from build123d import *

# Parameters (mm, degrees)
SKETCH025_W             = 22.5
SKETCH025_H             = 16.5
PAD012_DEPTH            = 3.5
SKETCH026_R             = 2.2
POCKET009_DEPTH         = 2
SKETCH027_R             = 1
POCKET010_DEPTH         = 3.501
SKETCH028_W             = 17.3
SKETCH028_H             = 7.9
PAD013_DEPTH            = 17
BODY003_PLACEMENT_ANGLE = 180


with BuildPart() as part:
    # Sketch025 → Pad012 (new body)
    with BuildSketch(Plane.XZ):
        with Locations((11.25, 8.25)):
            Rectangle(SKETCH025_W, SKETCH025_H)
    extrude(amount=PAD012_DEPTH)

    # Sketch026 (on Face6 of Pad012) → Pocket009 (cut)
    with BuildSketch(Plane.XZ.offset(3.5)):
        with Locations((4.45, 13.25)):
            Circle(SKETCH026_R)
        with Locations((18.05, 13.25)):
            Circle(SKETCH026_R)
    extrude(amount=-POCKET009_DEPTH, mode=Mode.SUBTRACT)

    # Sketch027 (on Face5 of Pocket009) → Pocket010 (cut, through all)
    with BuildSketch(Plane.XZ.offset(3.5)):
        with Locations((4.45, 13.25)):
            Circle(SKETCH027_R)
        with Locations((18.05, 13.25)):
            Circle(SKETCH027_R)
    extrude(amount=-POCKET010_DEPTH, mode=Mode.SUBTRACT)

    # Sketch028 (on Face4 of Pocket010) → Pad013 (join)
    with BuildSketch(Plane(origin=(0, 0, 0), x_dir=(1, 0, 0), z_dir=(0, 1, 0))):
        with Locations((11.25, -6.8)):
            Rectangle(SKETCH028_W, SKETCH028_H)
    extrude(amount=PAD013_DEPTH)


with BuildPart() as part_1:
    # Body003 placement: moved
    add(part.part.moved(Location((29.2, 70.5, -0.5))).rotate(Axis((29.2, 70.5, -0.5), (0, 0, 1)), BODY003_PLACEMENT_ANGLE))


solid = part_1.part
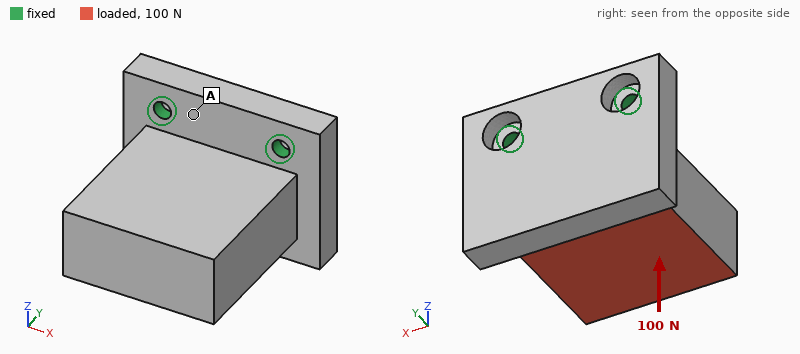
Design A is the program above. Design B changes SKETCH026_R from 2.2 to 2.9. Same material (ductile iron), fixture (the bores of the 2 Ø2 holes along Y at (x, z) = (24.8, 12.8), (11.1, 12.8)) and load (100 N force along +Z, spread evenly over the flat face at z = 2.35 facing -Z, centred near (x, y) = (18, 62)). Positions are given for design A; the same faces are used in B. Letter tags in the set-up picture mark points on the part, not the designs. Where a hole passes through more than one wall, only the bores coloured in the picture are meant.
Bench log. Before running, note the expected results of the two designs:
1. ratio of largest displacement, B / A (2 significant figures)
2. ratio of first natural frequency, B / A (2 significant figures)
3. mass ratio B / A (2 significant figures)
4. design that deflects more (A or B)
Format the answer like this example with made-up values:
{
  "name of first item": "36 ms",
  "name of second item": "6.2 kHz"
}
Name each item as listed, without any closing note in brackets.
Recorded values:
{
  "ratio of largest displacement, B / A": "1.1",
  "ratio of first natural frequency, B / A": "0.94",
  "mass ratio B / A": "0.99",
  "design that deflects more": "B"
}
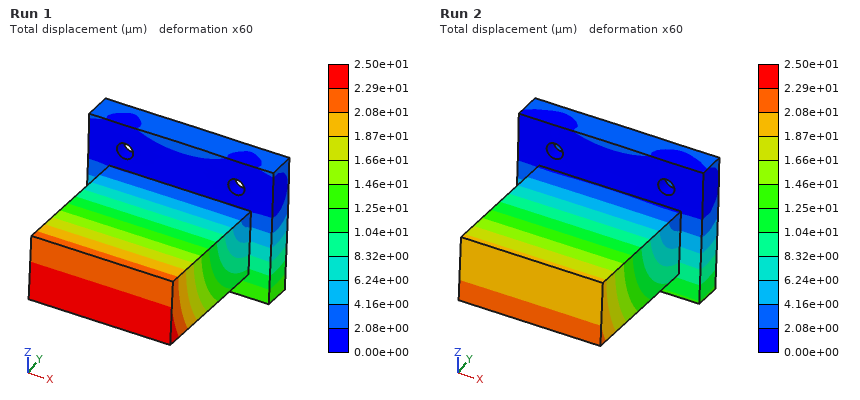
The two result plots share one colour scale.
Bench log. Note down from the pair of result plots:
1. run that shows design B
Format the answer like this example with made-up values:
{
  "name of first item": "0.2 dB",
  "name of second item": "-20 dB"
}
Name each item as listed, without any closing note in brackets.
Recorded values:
{
  "run that shows design B": "Run 1"
}
